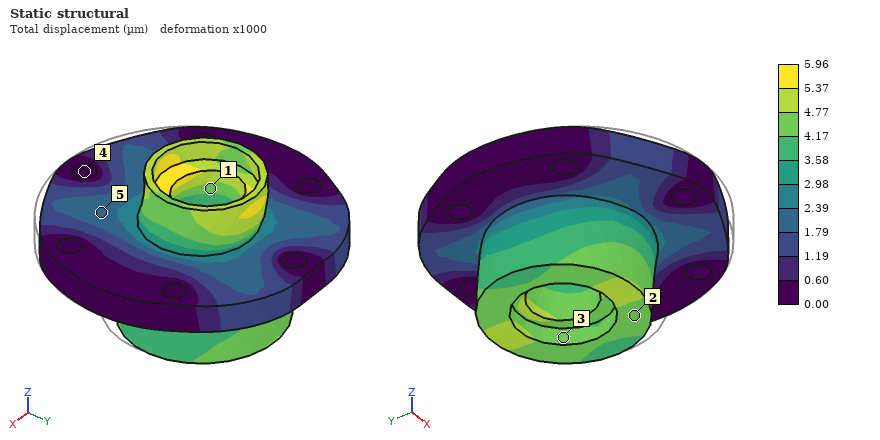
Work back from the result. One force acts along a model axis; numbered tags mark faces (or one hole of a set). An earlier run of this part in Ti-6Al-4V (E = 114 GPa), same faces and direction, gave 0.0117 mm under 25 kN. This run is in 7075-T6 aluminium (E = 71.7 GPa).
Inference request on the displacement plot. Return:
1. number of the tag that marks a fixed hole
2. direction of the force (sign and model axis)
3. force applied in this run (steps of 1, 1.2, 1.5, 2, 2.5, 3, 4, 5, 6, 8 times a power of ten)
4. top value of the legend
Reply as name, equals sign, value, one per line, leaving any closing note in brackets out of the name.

number of the tag that marks a fixed hole = 4
direction of the force = +Y
force applied in this run = 8 kN
top value of the legend = 5.96 µm
